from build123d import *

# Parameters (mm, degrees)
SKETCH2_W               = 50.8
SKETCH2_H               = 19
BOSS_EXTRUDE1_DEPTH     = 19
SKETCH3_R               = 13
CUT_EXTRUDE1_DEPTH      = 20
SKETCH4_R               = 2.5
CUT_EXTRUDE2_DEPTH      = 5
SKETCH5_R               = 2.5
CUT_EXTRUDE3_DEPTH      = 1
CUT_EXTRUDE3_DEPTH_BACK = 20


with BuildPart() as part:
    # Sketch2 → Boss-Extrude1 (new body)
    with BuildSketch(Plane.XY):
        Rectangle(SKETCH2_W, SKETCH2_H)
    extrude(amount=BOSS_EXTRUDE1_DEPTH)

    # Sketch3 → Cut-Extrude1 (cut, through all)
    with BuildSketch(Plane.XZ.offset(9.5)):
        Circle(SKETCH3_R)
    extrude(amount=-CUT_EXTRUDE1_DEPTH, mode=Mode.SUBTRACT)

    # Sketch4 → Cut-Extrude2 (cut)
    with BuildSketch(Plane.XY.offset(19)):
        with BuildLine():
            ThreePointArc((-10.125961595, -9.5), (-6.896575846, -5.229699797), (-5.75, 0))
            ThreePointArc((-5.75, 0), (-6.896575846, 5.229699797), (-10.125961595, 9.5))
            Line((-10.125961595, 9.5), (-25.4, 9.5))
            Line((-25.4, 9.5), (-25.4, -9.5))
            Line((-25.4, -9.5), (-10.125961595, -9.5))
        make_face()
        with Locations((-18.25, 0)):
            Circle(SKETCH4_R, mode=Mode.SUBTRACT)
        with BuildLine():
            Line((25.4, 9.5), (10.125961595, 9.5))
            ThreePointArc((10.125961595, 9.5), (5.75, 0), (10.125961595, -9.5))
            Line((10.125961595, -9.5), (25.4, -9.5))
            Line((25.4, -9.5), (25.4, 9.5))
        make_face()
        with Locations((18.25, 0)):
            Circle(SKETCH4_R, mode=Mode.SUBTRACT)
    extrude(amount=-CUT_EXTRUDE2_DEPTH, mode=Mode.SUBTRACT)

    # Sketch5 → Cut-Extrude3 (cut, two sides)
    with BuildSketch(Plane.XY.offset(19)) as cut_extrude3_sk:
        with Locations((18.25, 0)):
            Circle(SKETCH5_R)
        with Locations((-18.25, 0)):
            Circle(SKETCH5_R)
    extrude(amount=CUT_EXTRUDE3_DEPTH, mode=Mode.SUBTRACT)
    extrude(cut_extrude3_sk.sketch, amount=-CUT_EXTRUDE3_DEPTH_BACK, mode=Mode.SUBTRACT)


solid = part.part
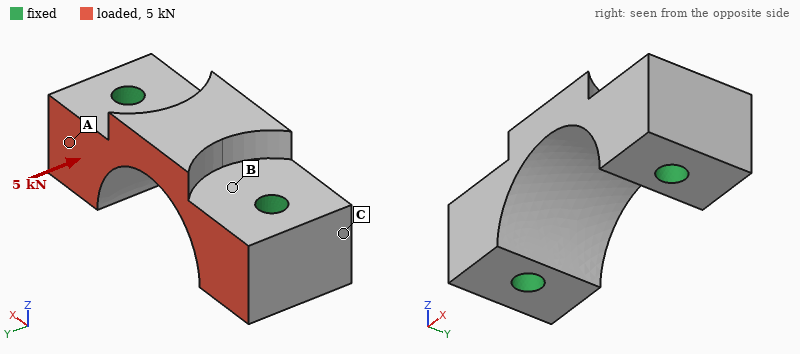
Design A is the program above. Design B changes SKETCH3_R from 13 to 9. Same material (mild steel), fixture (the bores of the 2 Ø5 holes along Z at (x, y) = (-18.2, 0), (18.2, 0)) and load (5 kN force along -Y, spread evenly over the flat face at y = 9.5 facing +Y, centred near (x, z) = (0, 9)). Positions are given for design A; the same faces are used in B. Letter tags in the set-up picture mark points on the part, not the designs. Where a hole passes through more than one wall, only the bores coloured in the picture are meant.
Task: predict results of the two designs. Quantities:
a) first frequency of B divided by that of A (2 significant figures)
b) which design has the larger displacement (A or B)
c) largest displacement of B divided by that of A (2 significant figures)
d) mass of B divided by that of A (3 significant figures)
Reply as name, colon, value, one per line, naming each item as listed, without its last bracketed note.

first frequency of B divided by that of A: 1.0
which design has the larger displacement: A
largest displacement of B divided by that of A: 0.76
mass of B divided by that of A: 1.28
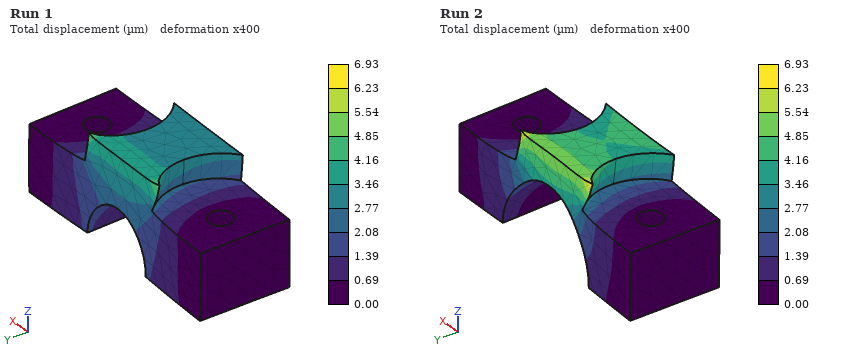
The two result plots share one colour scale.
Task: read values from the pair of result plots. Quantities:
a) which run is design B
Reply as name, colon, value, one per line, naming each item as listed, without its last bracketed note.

which run is design B: Run 1
